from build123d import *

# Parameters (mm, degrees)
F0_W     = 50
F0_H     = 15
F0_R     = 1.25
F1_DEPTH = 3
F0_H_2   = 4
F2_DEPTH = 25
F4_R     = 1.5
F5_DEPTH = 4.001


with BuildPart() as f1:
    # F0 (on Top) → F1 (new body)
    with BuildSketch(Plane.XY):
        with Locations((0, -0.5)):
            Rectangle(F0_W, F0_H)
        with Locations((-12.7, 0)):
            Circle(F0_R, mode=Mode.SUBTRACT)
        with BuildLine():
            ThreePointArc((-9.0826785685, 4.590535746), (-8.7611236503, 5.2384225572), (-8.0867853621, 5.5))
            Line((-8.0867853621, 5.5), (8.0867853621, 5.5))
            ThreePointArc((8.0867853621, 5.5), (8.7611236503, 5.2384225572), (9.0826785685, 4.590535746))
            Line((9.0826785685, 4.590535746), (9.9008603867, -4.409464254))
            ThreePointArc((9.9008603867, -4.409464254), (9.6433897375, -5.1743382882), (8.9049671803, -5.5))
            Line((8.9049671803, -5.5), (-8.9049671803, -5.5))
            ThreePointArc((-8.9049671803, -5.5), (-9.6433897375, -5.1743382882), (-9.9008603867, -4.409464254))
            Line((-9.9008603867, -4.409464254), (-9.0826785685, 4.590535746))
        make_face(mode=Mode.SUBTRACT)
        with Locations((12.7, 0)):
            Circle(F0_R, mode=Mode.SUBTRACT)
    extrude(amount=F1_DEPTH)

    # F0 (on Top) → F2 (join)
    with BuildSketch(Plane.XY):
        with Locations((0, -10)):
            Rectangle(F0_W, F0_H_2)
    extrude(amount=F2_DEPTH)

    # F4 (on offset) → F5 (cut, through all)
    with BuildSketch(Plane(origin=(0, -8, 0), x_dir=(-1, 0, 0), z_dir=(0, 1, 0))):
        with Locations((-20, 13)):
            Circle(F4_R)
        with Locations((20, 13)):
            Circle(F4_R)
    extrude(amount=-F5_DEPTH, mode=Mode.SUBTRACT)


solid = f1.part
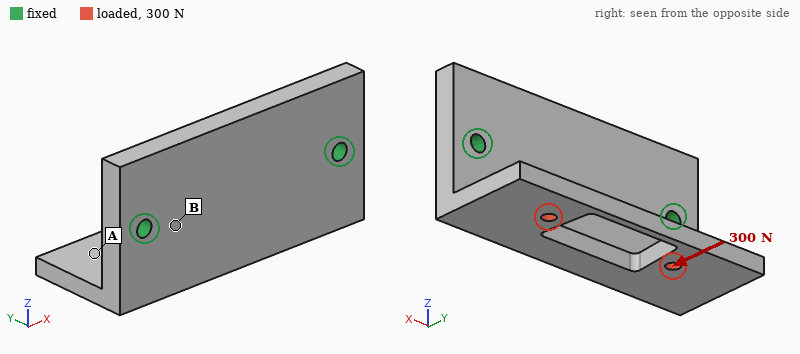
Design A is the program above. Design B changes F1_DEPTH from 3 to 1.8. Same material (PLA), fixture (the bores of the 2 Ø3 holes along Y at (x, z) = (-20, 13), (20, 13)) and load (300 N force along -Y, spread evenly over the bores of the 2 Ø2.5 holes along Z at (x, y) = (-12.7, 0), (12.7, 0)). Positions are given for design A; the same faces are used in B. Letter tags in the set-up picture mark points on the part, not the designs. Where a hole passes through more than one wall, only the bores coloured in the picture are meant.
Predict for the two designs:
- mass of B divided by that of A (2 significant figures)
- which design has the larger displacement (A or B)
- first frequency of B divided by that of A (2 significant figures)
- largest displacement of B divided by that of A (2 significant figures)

0.90
B
0.90
1.1
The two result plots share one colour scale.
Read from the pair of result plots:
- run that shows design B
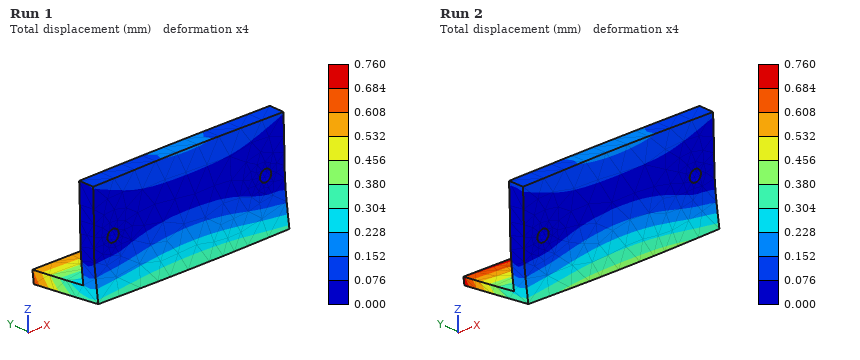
Run 2
